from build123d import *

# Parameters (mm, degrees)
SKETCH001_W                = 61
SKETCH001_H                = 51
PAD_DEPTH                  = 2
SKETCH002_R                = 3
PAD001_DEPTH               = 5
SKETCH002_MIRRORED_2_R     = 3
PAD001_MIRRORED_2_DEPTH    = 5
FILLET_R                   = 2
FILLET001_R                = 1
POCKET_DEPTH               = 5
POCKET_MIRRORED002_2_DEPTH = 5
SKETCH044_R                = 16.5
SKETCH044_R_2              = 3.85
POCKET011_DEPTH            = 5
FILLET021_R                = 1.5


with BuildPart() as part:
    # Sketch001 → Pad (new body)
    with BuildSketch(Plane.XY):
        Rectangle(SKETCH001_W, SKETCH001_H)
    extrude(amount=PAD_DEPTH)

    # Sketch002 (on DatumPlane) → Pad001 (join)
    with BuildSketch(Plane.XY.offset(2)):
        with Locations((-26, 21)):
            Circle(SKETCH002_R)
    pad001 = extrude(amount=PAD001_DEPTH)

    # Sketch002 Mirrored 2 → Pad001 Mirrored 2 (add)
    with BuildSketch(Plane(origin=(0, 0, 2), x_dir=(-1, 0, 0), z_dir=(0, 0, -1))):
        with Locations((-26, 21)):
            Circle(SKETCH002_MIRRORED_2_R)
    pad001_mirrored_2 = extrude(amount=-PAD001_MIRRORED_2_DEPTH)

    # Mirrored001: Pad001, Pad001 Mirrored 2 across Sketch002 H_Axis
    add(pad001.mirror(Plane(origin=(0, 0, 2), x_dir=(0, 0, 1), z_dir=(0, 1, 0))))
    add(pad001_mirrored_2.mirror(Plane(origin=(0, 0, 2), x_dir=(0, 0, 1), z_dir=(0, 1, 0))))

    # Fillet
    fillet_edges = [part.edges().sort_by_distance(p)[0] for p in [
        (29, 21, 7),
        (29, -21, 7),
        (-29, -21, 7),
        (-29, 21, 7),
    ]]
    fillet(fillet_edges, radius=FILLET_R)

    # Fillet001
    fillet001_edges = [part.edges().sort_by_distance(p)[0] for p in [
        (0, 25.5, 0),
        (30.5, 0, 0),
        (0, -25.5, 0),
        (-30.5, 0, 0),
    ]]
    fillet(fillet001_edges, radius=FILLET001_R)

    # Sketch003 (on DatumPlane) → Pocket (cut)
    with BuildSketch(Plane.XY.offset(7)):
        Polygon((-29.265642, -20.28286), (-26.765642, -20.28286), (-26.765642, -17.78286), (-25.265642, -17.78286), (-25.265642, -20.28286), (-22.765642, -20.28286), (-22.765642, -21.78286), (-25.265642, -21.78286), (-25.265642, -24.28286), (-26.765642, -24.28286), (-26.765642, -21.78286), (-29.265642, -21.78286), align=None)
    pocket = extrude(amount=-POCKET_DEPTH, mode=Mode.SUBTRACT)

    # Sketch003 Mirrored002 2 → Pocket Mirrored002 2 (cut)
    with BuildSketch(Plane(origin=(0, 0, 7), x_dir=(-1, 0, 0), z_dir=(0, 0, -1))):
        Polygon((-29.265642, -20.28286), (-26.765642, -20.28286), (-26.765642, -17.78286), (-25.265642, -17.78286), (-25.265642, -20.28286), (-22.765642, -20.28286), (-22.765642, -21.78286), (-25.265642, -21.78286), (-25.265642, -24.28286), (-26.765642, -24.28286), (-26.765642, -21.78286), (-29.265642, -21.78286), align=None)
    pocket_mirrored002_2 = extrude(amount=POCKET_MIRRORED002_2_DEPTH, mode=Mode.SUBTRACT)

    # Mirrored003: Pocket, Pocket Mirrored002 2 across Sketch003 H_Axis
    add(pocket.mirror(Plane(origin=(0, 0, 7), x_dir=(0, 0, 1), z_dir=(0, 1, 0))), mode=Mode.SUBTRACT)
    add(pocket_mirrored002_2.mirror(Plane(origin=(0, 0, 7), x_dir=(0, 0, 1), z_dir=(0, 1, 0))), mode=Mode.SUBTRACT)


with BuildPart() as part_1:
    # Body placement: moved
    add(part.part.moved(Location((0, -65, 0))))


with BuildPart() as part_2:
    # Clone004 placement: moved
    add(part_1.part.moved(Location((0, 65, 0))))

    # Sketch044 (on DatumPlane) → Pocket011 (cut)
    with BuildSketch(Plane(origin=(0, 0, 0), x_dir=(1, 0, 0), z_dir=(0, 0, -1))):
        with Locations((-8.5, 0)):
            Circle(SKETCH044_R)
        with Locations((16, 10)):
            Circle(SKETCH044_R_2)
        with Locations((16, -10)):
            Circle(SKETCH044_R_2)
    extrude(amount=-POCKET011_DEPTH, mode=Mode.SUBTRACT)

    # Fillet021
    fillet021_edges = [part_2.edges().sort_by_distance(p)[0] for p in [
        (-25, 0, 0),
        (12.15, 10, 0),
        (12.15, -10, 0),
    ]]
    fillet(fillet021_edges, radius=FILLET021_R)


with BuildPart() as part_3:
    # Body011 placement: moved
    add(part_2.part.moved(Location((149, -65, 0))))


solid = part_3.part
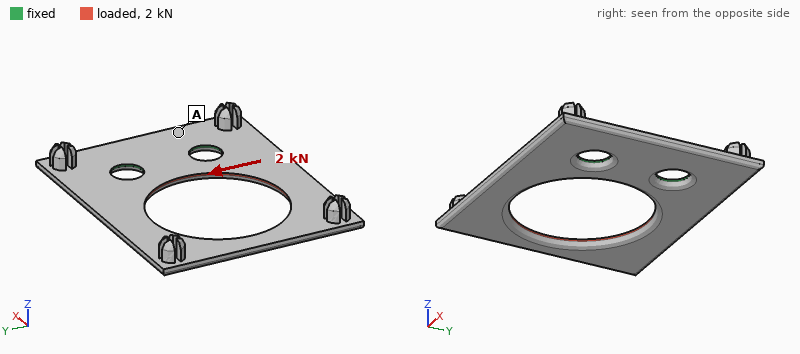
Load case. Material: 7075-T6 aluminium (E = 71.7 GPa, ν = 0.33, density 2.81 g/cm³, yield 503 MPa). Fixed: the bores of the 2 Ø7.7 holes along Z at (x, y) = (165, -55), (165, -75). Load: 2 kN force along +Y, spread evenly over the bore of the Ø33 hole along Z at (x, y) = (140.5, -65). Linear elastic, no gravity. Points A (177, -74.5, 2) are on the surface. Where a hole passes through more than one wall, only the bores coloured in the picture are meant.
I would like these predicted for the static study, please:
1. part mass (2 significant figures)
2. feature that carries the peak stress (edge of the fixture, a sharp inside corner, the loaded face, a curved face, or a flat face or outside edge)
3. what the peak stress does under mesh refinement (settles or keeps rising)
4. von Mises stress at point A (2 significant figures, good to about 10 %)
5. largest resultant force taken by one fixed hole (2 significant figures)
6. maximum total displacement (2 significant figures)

12 g
edge of the fixture
keeps rising
33 MPa
1.7 kN
0.44 mm
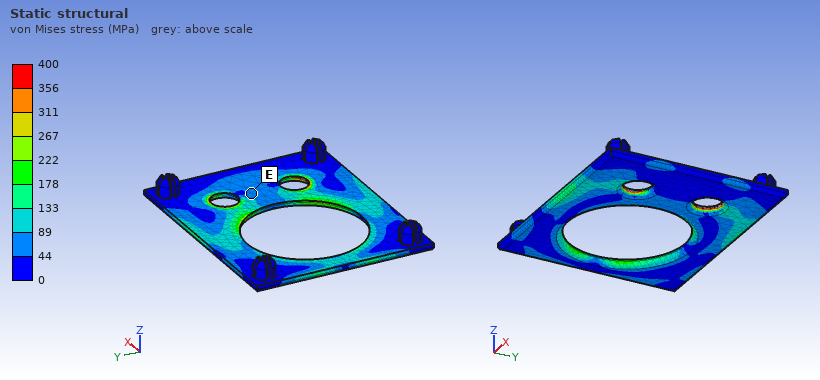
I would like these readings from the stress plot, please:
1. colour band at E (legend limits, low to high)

44 to 89 MPa
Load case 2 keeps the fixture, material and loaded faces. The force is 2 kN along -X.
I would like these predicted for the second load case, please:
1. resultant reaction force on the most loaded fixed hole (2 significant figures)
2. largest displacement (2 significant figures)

1.0 kN
0.83 mm
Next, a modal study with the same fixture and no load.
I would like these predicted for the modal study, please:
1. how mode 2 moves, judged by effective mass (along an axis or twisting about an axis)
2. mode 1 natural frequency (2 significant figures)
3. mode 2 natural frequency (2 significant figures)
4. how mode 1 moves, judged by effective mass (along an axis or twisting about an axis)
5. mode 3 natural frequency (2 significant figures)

twisting about X
610 Hz
1200 Hz
along Z
3200 Hz
